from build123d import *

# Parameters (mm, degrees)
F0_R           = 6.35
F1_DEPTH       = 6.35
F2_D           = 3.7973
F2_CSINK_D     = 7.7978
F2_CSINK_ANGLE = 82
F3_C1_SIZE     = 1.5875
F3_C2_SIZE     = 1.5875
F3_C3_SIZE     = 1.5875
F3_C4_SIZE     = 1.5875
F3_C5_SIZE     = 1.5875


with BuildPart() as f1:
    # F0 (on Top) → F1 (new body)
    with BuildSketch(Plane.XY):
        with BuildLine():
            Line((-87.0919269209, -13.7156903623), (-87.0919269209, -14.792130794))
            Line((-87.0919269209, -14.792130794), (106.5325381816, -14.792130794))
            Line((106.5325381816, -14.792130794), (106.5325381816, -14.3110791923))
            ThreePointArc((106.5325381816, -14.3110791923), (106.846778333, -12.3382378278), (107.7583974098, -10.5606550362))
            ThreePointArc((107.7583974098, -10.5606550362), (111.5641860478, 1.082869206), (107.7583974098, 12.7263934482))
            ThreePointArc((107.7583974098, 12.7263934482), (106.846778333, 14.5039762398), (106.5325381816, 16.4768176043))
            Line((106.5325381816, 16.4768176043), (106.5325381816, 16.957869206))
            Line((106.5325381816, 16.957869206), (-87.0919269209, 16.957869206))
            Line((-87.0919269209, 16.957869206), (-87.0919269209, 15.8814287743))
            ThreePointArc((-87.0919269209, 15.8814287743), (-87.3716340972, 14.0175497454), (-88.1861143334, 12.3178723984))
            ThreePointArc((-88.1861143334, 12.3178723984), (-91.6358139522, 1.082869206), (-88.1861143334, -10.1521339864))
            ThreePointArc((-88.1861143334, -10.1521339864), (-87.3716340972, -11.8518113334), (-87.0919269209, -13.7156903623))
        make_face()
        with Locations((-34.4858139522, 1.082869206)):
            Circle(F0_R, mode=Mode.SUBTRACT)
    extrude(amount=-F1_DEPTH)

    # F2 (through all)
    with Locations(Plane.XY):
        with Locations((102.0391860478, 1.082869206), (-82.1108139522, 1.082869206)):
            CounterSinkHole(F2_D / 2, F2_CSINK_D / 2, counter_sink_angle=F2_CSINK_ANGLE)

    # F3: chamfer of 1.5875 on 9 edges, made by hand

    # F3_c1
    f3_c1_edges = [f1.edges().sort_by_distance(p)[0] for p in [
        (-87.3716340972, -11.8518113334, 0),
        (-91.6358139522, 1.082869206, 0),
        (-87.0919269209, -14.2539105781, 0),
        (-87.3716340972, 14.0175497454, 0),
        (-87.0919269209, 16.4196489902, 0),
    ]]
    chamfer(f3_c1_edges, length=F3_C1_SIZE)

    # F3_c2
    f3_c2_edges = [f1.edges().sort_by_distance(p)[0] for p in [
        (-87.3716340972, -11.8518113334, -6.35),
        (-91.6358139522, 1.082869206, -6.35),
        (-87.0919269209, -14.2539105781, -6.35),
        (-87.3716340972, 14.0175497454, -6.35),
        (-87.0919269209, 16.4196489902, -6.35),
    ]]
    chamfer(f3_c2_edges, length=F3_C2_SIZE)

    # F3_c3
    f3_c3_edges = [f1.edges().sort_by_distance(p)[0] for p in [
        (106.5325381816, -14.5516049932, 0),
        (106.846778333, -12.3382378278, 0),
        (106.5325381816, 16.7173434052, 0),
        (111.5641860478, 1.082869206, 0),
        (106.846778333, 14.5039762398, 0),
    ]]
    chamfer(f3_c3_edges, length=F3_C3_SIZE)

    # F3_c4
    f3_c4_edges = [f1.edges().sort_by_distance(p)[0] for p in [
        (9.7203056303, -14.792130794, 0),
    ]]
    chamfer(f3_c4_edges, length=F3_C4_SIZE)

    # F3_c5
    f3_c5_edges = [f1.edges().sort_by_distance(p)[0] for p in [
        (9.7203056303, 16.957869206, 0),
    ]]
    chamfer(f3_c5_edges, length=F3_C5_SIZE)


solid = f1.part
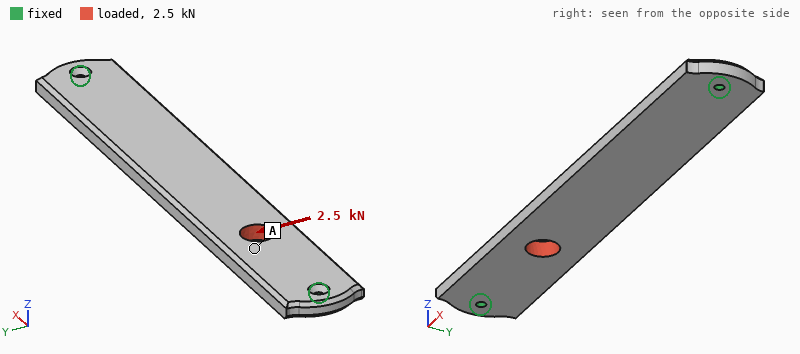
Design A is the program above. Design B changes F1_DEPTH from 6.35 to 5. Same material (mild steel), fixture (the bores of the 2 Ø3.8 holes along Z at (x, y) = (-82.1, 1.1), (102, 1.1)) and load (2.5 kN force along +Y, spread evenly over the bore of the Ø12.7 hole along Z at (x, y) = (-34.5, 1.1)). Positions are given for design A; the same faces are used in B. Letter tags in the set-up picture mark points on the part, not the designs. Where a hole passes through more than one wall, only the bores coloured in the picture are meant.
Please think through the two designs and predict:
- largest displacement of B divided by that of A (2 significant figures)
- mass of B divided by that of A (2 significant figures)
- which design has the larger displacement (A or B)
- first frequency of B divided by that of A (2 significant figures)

1.3
0.78
B
0.79
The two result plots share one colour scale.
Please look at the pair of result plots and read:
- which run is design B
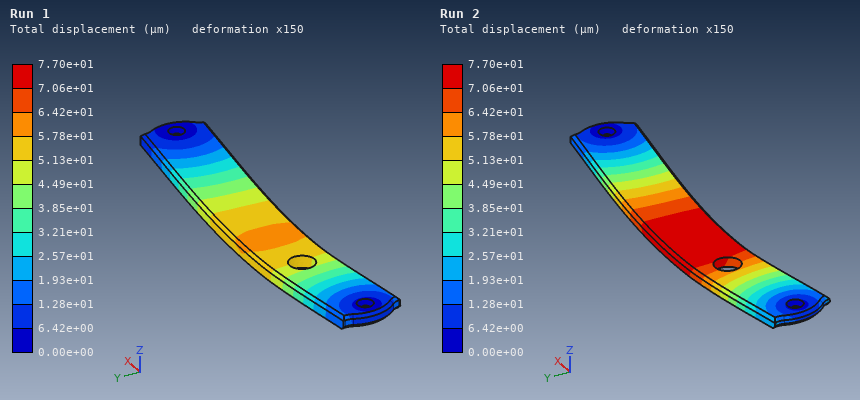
Run 2
